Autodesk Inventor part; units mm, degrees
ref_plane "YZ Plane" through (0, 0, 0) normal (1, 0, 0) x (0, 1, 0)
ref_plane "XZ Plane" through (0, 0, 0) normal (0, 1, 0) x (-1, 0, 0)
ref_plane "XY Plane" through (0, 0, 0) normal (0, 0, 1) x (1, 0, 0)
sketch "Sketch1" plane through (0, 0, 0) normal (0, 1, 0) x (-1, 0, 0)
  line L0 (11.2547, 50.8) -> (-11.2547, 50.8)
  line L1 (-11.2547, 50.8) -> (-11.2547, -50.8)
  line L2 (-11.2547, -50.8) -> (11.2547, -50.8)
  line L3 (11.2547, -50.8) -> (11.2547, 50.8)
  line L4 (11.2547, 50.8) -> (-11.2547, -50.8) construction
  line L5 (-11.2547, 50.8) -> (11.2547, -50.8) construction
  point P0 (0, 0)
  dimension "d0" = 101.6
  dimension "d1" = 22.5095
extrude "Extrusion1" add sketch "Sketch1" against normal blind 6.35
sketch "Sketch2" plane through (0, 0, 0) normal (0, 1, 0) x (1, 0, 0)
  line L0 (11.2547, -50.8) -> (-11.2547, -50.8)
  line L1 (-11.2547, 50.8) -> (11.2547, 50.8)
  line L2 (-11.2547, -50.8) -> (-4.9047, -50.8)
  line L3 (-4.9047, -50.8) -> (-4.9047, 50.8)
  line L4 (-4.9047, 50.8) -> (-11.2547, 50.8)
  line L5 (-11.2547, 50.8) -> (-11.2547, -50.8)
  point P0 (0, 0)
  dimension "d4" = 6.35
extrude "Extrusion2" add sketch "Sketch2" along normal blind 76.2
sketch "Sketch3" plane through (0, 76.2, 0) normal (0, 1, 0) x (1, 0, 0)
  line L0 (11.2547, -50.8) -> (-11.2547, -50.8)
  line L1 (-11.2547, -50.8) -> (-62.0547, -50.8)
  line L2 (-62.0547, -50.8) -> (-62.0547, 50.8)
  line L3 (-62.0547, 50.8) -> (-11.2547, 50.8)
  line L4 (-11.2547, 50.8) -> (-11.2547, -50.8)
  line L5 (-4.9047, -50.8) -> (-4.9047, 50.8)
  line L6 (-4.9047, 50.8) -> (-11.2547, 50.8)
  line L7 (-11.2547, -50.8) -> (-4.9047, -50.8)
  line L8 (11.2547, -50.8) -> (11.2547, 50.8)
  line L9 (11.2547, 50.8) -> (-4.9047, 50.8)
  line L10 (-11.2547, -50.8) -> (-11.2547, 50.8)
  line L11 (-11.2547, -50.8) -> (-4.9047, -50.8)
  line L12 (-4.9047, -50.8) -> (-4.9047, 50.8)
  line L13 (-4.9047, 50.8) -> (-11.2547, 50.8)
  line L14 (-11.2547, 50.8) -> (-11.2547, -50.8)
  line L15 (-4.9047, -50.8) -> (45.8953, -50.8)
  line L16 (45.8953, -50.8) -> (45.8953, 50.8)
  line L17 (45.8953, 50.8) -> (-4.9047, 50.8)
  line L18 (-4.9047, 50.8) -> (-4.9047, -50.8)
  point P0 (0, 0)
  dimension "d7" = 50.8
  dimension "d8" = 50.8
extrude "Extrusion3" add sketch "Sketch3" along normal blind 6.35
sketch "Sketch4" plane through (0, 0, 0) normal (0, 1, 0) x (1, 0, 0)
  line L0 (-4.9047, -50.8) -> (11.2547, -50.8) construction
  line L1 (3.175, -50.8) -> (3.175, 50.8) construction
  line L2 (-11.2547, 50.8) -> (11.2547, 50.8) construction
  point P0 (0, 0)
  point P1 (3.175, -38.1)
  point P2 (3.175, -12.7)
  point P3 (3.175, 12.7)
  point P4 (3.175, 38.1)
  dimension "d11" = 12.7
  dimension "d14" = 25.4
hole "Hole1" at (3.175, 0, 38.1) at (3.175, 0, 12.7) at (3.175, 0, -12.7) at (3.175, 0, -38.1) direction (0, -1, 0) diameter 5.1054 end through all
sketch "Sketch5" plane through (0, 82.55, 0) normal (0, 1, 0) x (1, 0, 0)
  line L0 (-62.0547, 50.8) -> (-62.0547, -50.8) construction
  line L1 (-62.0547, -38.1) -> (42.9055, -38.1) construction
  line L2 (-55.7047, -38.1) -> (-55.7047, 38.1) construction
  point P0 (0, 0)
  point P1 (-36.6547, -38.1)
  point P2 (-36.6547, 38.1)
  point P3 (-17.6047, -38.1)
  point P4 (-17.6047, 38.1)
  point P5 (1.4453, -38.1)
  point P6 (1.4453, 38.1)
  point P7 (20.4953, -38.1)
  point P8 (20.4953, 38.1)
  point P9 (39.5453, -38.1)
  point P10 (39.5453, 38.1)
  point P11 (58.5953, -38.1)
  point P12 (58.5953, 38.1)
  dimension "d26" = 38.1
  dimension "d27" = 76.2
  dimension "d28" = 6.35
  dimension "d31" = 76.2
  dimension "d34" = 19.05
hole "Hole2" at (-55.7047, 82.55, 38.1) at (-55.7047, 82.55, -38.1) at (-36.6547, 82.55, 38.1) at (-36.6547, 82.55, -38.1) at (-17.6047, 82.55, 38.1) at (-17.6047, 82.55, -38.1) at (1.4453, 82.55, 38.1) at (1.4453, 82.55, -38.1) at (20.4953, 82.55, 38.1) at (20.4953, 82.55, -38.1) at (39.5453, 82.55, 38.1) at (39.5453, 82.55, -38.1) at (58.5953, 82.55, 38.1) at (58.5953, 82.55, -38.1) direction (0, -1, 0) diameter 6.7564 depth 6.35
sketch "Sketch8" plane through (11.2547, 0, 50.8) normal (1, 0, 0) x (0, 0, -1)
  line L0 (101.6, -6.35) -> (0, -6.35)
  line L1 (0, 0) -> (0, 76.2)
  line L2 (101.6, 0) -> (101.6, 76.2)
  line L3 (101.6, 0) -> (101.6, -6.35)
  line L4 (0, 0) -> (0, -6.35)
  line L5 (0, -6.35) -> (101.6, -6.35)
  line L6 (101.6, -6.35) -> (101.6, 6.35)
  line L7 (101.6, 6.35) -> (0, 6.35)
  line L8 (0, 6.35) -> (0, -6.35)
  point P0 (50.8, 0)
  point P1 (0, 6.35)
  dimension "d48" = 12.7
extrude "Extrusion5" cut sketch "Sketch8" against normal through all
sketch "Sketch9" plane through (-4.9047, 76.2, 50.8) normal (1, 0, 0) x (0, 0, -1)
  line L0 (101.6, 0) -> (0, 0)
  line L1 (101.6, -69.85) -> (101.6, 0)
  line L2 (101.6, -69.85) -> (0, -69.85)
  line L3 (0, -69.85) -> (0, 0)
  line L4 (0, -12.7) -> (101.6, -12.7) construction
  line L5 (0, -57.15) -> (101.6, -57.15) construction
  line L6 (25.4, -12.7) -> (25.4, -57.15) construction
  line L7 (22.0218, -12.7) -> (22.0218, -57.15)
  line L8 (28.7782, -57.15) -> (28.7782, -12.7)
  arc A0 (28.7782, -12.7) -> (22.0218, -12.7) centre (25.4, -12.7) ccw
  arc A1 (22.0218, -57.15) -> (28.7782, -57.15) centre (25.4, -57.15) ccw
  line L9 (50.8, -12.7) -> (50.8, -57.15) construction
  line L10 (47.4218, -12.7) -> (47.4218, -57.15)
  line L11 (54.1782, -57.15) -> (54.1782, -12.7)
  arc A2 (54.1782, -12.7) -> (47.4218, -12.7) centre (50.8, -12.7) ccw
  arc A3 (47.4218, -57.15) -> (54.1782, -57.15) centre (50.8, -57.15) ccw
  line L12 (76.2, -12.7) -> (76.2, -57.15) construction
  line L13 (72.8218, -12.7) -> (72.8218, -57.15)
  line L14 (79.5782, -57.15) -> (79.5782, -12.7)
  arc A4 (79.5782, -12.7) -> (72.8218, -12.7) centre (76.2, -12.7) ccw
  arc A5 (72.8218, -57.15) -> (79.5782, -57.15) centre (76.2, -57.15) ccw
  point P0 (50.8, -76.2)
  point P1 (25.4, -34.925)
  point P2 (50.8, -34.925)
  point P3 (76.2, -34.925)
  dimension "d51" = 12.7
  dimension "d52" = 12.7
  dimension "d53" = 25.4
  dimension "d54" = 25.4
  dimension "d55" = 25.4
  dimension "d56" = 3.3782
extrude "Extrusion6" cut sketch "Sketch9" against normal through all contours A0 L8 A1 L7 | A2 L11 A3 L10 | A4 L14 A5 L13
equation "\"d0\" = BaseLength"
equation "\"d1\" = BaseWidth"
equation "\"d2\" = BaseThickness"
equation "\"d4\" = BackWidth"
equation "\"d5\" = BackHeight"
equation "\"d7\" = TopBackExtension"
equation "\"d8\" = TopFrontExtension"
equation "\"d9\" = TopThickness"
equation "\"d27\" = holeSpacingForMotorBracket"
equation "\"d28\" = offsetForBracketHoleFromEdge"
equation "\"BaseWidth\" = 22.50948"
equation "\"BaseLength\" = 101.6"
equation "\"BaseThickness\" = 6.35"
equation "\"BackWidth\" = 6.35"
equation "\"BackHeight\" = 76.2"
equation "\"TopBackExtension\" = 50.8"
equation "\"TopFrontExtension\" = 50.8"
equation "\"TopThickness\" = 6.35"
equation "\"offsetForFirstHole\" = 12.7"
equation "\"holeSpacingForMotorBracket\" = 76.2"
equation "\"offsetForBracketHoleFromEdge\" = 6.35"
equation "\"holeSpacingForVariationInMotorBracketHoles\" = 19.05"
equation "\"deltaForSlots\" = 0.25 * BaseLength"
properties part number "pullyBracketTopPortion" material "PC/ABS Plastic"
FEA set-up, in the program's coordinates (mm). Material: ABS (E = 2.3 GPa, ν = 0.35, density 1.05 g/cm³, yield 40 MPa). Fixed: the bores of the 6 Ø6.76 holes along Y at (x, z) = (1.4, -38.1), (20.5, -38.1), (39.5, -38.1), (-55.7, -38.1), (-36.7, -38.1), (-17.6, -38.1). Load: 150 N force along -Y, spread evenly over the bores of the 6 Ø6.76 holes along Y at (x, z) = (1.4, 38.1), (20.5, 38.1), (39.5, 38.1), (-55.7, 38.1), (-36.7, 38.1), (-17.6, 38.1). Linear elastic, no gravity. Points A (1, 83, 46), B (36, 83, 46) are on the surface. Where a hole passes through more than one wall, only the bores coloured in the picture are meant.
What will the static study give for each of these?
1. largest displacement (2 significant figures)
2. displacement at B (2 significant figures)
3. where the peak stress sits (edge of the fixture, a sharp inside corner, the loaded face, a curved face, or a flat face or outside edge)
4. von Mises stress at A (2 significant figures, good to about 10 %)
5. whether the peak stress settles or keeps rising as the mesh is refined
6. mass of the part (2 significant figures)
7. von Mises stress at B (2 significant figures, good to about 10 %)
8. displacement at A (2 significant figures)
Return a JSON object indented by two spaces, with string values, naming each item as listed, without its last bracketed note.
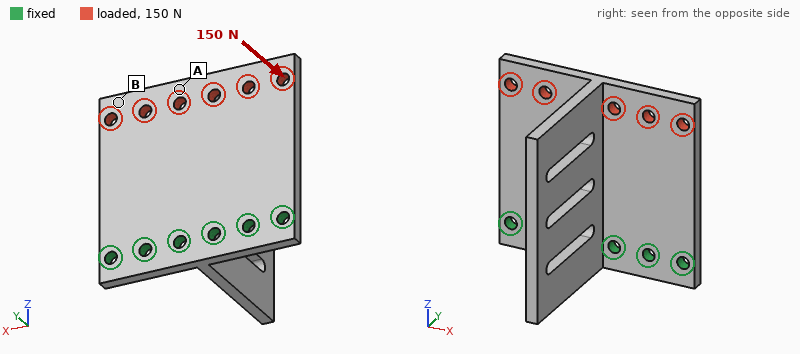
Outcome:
{
  "largest displacement": "1.7 mm",
  "displacement at B": "1.6 mm",
  "where the peak stress sits": "edge of the fixture",
  "von Mises stress at A": "3.6 MPa",
  "whether the peak stress settles or keeps rising as the mesh is refined": "keeps rising",
  "mass of the part": "110 g",
  "von Mises stress at B": "1.0 MPa",
  "displacement at A": "1.3 mm"
}
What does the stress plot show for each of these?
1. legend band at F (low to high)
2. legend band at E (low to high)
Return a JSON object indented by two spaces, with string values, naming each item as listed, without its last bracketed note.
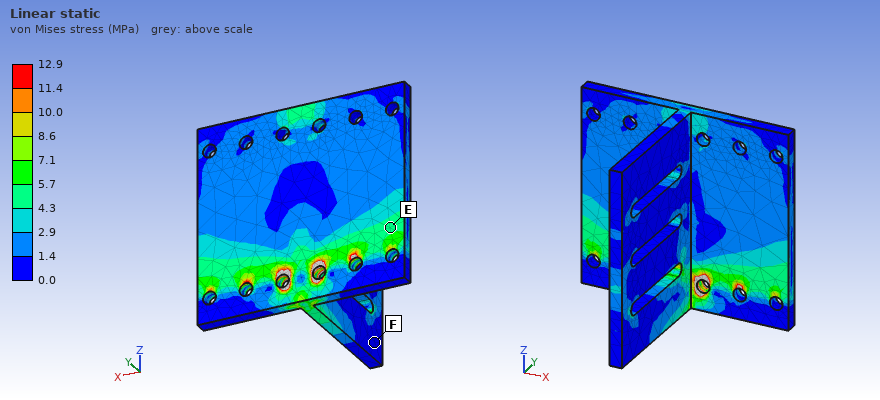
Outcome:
{
  "legend band at F": "0.0 to 1.4 MPa",
  "legend band at E": "4.3 to 5.7 MPa"
}
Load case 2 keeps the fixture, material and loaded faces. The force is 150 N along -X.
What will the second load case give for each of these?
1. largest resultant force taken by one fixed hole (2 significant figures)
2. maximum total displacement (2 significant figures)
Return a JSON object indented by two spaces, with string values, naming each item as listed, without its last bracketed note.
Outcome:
{
  "largest resultant force taken by one fixed hole": "92 N",
  "maximum total displacement": "45 µm"
}
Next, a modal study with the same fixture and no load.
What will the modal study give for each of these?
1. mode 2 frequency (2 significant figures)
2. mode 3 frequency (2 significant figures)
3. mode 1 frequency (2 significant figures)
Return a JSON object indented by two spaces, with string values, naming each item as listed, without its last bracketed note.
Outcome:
{
  "mode 2 frequency": "250 Hz",
  "mode 3 frequency": "440 Hz",
  "mode 1 frequency": "240 Hz"
}
